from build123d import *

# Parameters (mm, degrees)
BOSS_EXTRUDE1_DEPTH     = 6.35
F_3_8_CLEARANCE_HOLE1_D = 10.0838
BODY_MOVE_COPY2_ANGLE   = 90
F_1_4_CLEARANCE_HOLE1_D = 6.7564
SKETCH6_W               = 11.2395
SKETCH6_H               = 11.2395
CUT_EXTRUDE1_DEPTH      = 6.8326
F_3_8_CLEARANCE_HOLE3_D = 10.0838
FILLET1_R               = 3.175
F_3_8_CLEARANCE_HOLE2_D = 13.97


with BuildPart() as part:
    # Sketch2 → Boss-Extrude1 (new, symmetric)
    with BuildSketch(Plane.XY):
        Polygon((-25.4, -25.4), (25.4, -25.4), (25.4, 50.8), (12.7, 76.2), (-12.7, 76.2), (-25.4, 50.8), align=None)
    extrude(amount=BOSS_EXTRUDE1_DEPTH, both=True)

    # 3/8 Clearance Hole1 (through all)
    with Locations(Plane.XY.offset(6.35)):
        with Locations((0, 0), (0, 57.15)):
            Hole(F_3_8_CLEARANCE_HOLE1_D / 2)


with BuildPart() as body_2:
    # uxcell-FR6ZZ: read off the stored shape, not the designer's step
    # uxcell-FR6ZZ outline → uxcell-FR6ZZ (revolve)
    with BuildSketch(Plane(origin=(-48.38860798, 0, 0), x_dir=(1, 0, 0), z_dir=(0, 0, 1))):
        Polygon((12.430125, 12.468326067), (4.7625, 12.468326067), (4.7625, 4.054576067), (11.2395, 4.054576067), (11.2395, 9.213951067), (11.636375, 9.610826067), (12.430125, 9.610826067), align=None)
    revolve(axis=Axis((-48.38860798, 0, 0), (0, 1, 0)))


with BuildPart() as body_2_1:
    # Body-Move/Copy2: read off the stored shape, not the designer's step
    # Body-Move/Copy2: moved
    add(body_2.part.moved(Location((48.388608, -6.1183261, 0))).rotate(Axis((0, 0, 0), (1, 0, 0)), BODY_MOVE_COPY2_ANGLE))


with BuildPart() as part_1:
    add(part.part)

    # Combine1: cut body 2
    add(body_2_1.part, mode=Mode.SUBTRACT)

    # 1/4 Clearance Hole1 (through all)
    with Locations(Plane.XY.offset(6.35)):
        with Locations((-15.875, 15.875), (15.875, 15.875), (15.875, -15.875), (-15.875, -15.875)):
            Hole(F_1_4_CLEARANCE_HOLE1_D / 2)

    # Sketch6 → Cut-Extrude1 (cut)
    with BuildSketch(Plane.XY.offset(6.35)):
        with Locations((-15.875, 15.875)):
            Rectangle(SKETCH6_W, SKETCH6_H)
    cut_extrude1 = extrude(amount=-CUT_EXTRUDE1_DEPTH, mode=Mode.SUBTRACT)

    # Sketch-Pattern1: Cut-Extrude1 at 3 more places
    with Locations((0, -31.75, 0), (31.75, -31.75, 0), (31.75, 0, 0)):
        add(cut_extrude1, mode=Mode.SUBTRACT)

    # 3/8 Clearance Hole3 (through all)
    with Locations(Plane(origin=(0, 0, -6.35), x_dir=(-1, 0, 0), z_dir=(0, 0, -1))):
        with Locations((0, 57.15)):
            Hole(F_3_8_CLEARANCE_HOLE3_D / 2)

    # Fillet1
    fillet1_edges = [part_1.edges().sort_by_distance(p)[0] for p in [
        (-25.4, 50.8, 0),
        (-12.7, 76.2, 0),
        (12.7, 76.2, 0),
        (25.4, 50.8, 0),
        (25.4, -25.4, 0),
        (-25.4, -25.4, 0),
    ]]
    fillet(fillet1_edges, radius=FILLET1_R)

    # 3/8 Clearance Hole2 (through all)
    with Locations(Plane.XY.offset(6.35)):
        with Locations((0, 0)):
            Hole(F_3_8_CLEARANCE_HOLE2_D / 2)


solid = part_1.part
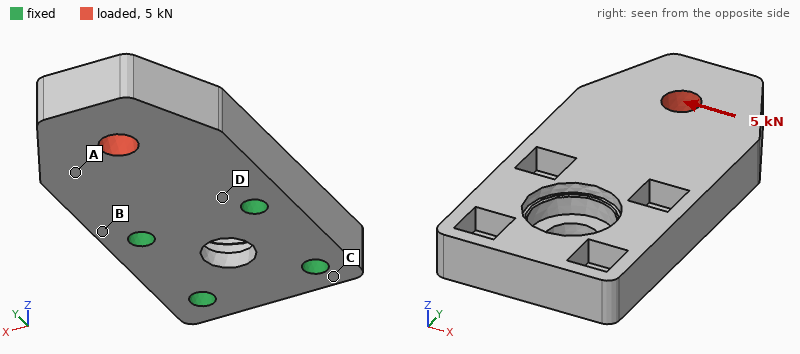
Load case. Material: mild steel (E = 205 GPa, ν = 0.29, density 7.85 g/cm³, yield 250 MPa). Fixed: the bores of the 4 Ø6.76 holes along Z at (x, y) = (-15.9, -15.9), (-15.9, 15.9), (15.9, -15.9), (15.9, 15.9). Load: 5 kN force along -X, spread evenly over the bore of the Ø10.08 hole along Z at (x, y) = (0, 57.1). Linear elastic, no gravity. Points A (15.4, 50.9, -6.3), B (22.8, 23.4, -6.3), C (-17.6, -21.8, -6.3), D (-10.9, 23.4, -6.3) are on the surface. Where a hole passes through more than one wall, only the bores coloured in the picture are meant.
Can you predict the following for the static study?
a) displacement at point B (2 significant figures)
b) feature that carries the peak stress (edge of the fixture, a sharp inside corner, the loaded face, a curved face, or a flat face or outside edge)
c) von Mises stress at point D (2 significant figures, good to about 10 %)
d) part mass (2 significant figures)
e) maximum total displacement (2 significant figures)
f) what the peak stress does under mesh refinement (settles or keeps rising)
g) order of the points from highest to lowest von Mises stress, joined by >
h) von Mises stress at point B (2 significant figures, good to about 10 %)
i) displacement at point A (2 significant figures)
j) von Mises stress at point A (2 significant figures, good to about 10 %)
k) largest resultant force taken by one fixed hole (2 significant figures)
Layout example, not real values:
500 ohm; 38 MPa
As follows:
3.1 µm; edge of the fixture; 42 MPa; 410 g; 17 µm; keeps rising; D > B > A > C; 28 MPa; 11 µm; 15 MPa; 5.5 kN
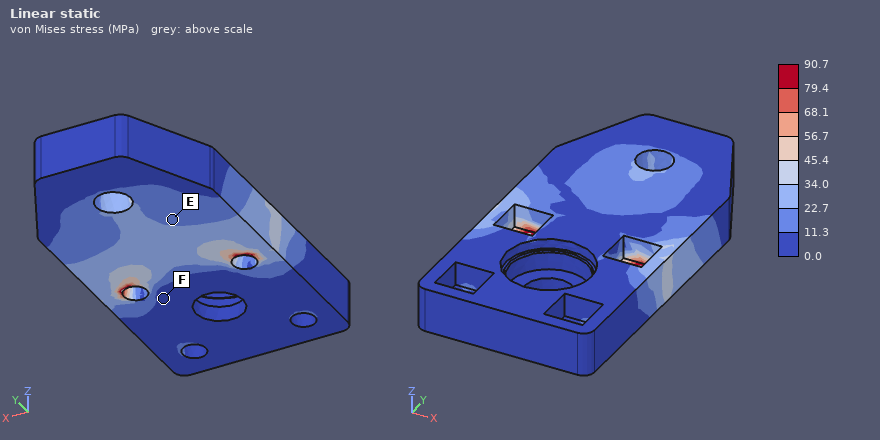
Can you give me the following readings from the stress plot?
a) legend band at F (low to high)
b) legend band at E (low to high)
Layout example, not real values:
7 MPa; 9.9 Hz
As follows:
0.0 to 11.3 MPa; 11.3 to 22.7 MPa
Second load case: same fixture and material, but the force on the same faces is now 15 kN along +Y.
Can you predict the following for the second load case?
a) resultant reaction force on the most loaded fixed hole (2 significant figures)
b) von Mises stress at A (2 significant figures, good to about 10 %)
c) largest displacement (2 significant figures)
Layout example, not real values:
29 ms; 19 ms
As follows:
6.2 kN; 21 MPa; 32 µm
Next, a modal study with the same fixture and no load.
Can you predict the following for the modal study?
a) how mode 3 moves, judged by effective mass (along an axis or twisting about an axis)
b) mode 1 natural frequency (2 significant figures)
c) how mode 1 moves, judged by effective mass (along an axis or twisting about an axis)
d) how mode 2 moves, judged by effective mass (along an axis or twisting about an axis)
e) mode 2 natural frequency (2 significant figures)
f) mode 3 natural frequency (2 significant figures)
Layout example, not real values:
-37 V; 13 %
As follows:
along X; 2400 Hz; along Z; along X; 7600 Hz; 8500 Hz
